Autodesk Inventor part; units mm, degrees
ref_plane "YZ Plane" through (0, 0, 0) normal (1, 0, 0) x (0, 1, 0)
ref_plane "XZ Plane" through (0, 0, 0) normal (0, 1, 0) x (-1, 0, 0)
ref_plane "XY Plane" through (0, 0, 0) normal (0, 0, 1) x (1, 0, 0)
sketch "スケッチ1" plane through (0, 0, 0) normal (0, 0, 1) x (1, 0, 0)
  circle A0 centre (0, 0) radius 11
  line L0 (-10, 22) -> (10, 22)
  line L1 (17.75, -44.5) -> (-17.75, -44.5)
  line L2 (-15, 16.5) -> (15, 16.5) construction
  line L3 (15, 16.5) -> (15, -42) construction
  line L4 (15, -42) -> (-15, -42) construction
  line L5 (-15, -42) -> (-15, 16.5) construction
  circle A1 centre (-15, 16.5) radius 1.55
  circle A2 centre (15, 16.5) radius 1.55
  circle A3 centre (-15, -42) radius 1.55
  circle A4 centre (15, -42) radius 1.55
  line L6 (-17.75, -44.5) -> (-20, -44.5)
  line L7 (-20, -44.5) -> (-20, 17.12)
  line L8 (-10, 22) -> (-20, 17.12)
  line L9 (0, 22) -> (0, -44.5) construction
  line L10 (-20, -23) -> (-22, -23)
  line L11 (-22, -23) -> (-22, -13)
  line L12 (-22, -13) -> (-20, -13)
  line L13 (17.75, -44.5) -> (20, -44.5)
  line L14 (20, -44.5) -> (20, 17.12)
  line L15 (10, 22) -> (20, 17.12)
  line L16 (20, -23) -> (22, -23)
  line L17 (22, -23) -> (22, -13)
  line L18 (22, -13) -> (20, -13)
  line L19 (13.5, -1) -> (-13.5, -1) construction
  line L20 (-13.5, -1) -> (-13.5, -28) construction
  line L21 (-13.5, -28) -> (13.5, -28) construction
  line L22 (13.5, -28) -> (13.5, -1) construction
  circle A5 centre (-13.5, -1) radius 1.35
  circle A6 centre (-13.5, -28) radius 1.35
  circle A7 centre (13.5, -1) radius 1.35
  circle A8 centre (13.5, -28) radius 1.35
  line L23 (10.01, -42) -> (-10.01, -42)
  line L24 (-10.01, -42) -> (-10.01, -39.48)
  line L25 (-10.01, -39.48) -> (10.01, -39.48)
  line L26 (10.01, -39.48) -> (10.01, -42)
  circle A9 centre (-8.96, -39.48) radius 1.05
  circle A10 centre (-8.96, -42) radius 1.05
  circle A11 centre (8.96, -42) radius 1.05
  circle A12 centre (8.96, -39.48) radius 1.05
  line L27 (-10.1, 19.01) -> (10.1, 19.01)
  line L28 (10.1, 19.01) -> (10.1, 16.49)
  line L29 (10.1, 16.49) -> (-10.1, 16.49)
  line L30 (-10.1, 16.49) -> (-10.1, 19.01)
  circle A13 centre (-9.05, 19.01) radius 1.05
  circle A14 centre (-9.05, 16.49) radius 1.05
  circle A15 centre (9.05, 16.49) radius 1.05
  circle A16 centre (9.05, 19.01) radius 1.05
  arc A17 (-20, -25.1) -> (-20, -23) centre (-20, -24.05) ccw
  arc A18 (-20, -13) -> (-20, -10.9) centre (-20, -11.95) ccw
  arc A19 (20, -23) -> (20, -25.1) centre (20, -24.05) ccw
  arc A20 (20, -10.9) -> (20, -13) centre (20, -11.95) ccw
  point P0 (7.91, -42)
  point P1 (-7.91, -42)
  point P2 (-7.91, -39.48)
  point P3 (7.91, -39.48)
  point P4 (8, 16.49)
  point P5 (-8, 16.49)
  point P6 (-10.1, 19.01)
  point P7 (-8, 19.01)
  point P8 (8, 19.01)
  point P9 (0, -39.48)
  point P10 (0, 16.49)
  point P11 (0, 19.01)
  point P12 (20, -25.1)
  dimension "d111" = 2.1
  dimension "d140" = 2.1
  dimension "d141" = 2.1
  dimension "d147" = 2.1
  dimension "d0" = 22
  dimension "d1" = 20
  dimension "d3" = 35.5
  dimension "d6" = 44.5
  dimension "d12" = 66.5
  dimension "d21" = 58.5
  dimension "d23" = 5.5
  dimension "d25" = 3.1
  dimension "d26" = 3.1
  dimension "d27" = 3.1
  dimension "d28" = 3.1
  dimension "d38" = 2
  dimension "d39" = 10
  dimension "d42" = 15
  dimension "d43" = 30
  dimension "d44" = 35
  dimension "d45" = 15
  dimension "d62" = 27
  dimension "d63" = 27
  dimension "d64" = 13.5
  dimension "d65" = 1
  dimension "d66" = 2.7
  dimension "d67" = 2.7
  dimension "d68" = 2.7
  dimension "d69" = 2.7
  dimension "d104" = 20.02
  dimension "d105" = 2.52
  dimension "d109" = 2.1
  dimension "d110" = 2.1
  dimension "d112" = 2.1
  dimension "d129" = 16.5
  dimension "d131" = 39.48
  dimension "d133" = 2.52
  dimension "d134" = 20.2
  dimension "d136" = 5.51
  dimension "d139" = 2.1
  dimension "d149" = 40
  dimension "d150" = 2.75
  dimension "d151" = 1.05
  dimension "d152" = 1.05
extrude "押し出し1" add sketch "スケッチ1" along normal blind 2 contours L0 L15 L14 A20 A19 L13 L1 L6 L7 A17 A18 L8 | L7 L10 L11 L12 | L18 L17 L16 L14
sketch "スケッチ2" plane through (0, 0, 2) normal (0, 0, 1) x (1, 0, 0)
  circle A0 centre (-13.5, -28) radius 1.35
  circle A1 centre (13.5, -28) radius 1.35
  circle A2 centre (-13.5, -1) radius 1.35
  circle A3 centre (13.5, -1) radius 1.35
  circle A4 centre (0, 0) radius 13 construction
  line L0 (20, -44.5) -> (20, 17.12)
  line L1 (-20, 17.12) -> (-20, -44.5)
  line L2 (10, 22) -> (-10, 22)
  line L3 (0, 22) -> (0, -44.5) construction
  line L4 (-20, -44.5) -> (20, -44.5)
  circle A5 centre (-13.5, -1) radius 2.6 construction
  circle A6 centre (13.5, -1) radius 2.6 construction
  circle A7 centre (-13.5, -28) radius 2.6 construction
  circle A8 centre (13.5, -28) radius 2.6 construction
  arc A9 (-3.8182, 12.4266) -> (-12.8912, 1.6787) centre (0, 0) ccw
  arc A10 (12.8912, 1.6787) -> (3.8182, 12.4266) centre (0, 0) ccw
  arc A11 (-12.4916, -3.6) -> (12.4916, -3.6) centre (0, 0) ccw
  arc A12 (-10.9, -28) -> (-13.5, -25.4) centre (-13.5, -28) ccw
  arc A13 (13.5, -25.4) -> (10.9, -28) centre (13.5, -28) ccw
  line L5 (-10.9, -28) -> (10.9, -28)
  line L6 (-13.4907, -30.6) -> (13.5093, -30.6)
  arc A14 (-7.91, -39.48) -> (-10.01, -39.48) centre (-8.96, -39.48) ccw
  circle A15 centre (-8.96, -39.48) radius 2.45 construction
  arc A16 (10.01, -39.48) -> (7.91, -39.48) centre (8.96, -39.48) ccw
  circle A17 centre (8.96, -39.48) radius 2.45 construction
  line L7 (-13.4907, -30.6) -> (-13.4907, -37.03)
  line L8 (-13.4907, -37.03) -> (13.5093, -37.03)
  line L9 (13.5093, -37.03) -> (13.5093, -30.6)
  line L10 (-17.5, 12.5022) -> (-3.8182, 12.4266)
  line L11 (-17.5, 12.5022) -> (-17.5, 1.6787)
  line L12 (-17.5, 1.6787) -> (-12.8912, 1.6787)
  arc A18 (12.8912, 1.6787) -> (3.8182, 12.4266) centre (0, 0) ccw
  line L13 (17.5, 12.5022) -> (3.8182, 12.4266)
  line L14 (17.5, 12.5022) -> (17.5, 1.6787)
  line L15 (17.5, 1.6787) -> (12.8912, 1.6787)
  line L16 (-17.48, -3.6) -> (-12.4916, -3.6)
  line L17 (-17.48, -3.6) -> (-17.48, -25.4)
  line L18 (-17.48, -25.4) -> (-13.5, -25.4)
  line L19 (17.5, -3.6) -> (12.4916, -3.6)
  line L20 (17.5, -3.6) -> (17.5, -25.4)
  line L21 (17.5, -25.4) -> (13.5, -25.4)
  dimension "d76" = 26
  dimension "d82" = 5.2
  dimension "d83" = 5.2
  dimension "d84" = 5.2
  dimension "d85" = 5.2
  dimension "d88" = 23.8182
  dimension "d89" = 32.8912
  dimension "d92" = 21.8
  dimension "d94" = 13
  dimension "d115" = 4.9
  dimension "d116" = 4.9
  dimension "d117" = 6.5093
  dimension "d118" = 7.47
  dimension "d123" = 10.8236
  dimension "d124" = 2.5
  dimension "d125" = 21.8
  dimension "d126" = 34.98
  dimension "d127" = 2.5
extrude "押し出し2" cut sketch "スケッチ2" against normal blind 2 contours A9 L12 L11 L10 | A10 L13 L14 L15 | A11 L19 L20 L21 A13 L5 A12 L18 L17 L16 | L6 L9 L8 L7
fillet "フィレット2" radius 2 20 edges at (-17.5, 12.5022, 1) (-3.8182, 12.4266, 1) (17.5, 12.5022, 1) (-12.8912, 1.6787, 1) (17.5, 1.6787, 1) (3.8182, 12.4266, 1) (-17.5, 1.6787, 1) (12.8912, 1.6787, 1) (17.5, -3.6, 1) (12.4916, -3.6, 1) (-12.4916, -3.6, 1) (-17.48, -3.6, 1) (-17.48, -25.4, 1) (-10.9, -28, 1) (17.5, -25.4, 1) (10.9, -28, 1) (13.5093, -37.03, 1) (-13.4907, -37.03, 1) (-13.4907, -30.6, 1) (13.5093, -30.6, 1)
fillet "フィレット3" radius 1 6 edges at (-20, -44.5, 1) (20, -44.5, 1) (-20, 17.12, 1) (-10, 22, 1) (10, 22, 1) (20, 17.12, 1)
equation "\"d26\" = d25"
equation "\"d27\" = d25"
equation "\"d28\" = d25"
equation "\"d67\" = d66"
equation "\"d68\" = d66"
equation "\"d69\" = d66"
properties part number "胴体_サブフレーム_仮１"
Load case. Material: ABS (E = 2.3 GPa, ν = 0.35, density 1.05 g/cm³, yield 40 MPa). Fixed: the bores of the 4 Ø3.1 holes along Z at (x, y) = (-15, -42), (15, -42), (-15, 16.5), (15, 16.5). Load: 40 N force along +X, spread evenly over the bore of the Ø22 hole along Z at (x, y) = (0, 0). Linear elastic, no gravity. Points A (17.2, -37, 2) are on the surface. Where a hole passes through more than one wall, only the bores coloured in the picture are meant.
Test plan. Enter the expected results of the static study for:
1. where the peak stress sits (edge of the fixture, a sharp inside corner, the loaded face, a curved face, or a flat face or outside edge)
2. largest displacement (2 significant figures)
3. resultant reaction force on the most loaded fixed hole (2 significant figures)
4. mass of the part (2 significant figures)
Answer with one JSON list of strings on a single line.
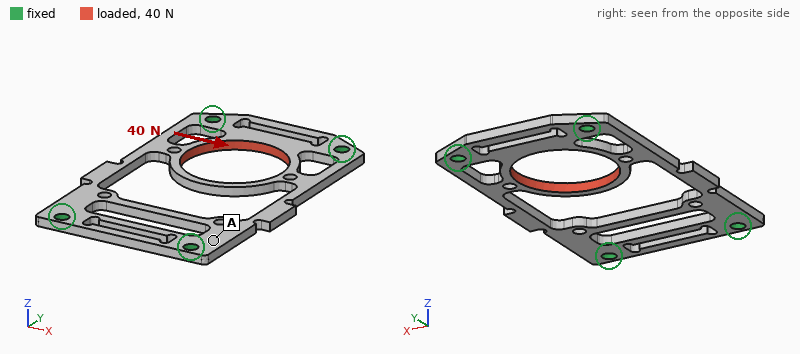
["a curved face", "0.21 mm", "21 N", "2.4 g"]
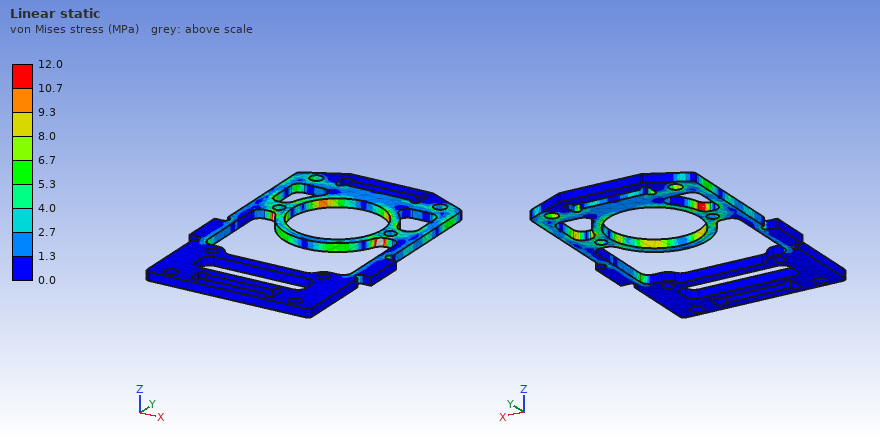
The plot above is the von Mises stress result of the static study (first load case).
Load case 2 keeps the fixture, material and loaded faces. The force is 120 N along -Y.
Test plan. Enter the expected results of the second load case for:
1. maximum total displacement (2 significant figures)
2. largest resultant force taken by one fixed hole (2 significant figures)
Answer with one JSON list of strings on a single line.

["0.32 mm", "53 N"]
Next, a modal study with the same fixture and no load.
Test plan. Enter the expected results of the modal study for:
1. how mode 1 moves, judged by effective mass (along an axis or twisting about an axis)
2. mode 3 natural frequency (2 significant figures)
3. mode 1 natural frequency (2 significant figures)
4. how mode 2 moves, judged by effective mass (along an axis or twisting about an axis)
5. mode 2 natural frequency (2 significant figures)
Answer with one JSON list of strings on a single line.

["along Z", "1400 Hz", "750 Hz", "twisting about Y", "1000 Hz"]
